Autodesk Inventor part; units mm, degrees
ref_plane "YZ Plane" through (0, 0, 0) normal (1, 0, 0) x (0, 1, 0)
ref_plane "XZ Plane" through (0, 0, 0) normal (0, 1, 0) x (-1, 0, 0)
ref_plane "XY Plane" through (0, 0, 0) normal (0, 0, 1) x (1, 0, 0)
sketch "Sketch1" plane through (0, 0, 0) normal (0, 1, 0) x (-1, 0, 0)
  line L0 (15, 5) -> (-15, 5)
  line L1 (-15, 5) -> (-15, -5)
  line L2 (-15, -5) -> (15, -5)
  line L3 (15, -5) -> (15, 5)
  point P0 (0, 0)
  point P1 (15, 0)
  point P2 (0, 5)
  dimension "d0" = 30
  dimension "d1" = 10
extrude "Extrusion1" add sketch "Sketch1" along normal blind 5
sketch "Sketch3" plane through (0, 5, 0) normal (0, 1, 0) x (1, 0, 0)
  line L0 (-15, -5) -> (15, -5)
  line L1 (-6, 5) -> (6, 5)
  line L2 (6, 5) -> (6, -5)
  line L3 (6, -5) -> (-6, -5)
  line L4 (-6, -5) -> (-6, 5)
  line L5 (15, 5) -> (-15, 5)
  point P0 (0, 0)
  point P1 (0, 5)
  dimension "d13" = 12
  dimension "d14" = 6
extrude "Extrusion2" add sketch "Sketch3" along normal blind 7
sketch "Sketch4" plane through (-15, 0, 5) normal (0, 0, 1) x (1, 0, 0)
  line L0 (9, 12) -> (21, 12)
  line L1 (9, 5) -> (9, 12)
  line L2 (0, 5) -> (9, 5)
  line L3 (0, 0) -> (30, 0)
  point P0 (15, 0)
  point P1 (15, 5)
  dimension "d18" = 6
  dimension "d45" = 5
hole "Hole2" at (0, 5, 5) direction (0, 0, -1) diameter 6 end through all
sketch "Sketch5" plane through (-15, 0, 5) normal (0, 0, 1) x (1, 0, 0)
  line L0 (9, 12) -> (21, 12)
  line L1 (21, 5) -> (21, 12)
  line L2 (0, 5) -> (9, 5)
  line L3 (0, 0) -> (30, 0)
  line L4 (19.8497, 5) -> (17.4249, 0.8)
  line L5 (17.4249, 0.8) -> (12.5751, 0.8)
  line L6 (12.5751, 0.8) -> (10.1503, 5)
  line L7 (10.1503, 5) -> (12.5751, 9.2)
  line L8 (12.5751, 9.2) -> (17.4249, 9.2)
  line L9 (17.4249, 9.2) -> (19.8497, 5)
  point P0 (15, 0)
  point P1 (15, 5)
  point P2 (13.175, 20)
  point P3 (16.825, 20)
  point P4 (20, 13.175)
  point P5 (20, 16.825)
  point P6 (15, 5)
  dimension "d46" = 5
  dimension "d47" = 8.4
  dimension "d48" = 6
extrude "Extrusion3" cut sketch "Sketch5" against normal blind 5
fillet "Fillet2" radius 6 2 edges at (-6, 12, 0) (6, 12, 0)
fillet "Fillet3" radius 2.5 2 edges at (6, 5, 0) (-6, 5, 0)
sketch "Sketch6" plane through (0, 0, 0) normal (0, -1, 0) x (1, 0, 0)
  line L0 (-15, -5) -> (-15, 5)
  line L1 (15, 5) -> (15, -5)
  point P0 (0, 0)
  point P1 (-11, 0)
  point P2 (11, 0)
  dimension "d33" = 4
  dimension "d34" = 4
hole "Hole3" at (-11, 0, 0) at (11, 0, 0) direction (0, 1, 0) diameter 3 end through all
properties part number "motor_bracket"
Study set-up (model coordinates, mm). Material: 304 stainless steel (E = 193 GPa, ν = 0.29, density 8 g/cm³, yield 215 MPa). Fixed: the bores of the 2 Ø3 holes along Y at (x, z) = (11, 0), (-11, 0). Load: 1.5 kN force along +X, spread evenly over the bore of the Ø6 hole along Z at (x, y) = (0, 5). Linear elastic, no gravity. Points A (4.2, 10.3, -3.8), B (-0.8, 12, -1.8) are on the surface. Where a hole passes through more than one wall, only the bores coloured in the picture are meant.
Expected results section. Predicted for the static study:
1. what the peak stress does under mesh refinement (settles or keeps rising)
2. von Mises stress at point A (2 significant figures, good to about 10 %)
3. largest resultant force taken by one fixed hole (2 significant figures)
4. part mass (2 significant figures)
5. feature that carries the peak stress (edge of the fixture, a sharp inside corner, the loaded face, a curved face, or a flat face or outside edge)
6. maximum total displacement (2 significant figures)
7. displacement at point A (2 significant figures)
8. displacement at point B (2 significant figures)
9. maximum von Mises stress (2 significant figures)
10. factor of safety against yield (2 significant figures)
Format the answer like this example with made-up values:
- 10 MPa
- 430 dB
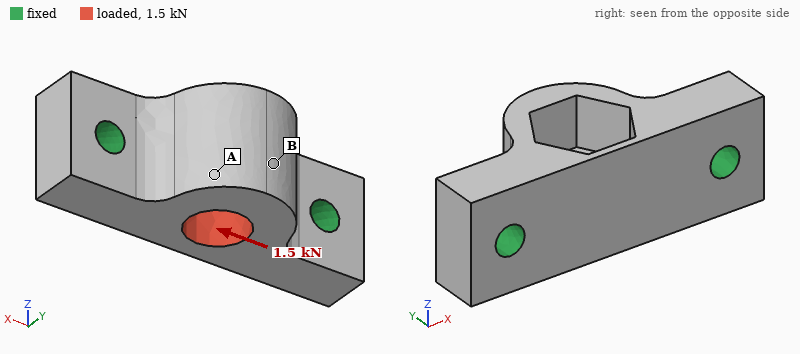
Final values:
- settles
- 16 MPa
- 780 N
- 14 g
- a curved face
- 2.4 µm
- 2.0 µm
- 1.5 µm
- 61 MPa
- 3.5
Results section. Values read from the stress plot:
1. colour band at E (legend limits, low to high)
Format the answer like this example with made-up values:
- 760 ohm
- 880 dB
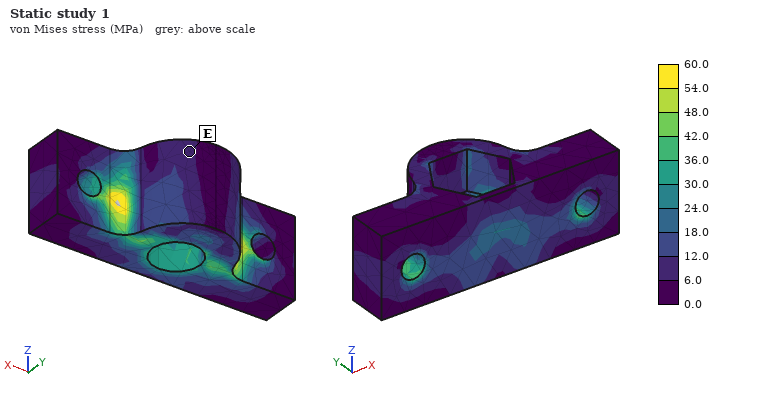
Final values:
- 6.0 to 12.0 MPa
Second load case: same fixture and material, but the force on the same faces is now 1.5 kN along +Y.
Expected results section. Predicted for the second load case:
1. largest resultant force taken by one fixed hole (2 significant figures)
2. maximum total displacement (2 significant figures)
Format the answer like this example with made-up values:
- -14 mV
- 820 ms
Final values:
- 750 N
- 6.9 µm
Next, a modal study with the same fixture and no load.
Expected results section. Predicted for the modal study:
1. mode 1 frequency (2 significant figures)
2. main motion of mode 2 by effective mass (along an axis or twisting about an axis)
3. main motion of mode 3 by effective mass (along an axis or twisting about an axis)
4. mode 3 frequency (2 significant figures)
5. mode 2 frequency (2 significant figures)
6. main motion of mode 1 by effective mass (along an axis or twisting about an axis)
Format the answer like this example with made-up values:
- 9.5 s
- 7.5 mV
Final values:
- 27 kHz
- along Y
- along X
- 50 kHz
- 44 kHz
- along Z
